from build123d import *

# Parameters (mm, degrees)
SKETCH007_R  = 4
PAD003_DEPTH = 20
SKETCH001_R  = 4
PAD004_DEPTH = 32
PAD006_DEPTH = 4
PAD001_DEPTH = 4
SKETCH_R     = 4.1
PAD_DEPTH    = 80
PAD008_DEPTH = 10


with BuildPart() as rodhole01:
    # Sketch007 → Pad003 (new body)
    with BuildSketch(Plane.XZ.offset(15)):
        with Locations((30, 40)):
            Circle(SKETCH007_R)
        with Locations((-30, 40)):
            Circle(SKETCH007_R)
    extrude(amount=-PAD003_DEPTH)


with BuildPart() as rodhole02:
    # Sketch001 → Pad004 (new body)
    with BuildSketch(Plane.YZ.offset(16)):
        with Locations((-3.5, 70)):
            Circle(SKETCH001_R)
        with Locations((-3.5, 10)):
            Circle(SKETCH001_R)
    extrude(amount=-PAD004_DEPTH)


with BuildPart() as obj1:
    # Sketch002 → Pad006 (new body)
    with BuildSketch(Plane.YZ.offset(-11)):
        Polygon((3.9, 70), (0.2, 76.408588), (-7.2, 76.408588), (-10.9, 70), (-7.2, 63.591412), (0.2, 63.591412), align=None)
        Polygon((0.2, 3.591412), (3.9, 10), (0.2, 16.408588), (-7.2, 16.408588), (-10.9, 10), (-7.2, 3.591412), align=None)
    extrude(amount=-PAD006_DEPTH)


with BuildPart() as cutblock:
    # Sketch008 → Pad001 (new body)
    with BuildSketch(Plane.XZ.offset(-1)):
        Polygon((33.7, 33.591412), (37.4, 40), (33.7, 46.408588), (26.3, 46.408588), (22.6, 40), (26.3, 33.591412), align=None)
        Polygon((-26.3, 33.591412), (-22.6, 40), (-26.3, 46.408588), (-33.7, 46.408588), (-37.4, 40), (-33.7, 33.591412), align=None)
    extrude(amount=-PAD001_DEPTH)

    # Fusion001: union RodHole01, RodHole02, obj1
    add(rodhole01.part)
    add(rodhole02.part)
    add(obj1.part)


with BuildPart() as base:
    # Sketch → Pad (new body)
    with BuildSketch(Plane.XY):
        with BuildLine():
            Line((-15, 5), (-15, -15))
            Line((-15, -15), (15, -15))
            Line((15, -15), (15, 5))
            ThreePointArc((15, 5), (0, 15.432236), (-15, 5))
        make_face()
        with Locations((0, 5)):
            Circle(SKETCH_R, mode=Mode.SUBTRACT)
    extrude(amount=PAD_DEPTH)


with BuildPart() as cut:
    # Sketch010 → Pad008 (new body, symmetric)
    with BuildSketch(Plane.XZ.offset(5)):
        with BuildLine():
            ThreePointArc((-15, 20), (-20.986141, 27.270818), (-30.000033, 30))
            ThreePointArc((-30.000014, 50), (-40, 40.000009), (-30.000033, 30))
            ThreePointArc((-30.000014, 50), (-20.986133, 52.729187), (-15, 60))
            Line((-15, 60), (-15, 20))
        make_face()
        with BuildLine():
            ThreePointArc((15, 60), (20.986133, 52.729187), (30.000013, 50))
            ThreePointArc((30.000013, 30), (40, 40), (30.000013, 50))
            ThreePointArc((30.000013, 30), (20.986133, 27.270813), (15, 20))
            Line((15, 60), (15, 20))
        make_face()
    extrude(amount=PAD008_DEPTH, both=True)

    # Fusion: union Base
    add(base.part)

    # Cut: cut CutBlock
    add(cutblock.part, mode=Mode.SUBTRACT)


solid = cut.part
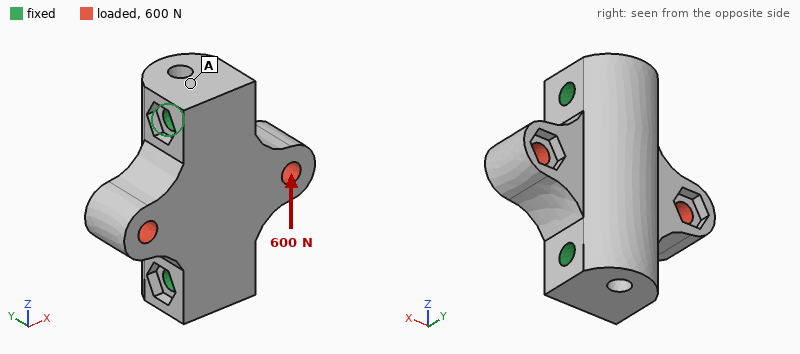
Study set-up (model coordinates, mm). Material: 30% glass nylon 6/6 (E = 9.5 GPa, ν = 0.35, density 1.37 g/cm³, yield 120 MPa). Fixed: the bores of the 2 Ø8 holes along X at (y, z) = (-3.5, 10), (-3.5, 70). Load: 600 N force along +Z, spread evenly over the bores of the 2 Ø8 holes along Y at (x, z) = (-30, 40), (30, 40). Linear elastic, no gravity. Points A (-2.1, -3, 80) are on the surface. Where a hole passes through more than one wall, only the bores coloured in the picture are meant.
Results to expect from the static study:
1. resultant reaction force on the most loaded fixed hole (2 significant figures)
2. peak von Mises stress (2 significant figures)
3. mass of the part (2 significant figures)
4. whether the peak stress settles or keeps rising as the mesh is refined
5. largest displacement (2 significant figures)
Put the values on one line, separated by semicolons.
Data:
300 N; 3.9 MPa; 110 g; settles; 10 µm
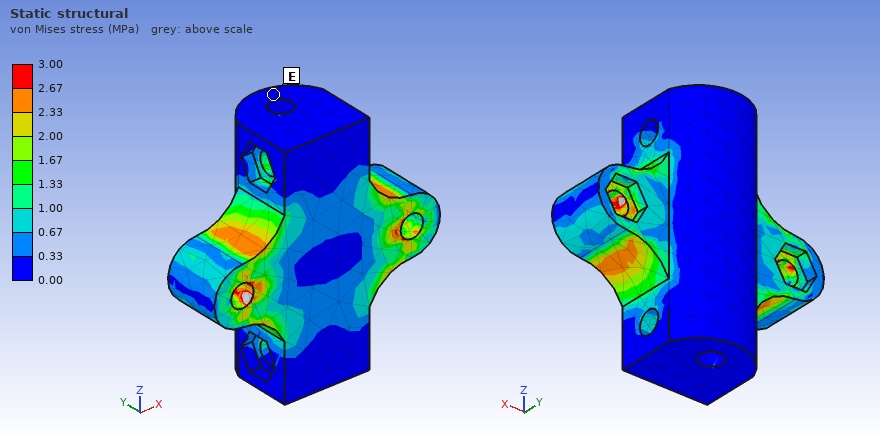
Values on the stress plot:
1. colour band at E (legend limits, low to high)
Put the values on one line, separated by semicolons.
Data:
0.00 to 0.33 MPa
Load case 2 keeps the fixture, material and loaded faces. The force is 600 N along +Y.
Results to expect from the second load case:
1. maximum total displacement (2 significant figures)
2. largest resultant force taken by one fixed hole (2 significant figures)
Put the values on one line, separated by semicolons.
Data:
25 µm; 310 N
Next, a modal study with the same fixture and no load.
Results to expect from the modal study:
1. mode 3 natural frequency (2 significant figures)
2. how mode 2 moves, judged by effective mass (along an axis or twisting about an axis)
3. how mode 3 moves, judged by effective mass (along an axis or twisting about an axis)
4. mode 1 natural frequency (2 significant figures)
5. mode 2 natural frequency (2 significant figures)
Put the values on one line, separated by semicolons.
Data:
8700 Hz; along Y; along X; 5200 Hz; 6200 Hz
